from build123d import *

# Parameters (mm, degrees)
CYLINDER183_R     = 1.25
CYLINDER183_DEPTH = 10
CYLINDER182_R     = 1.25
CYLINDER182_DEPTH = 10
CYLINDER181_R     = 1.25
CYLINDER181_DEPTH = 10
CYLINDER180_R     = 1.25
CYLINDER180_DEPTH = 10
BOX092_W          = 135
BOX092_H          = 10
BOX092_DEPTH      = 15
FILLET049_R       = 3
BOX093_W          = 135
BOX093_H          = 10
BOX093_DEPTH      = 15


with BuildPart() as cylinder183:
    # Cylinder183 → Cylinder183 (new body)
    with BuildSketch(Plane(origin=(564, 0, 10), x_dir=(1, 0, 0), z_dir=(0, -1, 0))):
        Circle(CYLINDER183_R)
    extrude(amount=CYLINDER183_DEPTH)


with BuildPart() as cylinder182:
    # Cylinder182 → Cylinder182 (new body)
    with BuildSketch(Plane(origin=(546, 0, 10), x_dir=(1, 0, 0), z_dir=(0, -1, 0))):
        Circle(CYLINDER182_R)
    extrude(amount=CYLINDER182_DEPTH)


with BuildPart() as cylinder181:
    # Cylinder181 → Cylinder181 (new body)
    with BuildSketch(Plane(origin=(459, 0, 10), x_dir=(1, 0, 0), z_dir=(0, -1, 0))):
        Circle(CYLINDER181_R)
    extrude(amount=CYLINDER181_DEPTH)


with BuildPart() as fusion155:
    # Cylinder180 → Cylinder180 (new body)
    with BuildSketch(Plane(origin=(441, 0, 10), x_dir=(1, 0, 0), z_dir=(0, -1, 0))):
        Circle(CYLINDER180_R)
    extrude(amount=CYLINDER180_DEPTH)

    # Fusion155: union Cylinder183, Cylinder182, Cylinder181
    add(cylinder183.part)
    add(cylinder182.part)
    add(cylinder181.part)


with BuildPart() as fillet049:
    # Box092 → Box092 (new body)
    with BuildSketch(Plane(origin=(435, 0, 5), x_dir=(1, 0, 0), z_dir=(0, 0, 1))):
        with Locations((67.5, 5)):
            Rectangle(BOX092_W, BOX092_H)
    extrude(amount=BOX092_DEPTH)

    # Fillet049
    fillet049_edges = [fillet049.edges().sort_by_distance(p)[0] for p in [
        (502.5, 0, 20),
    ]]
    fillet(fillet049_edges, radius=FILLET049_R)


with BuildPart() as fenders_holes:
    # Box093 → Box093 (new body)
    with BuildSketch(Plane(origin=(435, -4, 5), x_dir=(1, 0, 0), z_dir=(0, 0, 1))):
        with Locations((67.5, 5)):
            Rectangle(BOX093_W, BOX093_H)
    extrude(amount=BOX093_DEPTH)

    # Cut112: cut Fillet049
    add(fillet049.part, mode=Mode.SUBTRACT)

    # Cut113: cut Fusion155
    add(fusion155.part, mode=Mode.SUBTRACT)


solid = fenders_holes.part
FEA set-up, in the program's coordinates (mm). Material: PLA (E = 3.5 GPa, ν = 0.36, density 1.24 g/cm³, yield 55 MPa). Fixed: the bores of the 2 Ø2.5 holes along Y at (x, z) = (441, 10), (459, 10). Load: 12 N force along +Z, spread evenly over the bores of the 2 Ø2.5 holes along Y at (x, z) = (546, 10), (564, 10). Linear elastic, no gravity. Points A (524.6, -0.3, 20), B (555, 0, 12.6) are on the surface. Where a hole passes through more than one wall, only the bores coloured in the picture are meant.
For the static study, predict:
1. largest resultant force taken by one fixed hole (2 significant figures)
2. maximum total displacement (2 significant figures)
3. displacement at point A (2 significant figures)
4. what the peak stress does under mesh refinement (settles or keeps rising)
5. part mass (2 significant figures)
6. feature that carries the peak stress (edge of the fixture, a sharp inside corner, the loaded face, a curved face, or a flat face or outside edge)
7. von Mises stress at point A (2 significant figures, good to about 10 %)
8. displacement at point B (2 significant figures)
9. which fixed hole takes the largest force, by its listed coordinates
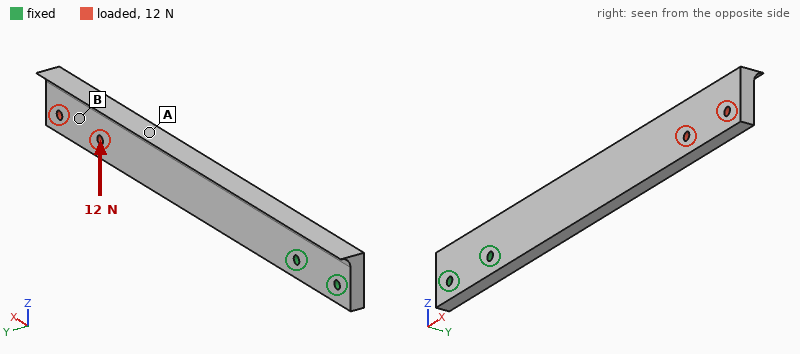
75 N
1.3 mm
0.63 mm
keeps rising
10 g
edge of the fixture
2.0 MPa
1.1 mm
(459, 10)
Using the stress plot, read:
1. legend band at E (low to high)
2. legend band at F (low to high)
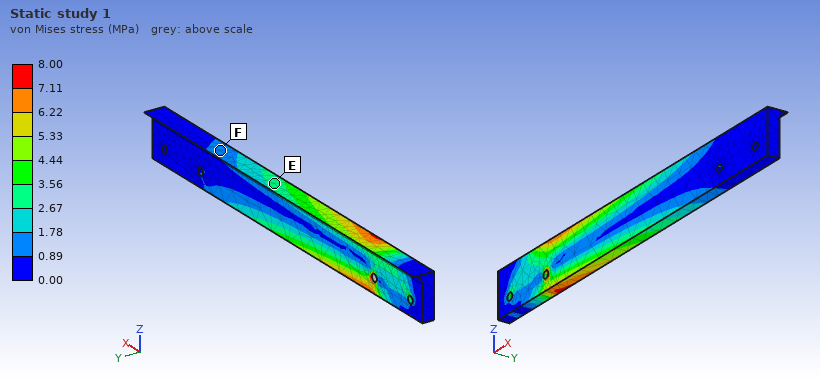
2.67 to 3.56 MPa
0.89 to 1.78 MPa
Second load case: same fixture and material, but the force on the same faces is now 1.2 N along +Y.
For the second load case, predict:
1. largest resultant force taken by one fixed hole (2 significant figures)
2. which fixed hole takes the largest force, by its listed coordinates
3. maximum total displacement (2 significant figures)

3.6 N
(459, 10)
1.4 mm
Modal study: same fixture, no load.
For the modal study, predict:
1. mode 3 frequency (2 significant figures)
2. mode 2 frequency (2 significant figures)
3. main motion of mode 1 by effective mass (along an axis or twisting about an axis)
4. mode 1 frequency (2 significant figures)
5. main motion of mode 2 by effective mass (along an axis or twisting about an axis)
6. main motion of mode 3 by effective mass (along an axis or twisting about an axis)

570 Hz
300 Hz
along Y
92 Hz
along Z
along Y
